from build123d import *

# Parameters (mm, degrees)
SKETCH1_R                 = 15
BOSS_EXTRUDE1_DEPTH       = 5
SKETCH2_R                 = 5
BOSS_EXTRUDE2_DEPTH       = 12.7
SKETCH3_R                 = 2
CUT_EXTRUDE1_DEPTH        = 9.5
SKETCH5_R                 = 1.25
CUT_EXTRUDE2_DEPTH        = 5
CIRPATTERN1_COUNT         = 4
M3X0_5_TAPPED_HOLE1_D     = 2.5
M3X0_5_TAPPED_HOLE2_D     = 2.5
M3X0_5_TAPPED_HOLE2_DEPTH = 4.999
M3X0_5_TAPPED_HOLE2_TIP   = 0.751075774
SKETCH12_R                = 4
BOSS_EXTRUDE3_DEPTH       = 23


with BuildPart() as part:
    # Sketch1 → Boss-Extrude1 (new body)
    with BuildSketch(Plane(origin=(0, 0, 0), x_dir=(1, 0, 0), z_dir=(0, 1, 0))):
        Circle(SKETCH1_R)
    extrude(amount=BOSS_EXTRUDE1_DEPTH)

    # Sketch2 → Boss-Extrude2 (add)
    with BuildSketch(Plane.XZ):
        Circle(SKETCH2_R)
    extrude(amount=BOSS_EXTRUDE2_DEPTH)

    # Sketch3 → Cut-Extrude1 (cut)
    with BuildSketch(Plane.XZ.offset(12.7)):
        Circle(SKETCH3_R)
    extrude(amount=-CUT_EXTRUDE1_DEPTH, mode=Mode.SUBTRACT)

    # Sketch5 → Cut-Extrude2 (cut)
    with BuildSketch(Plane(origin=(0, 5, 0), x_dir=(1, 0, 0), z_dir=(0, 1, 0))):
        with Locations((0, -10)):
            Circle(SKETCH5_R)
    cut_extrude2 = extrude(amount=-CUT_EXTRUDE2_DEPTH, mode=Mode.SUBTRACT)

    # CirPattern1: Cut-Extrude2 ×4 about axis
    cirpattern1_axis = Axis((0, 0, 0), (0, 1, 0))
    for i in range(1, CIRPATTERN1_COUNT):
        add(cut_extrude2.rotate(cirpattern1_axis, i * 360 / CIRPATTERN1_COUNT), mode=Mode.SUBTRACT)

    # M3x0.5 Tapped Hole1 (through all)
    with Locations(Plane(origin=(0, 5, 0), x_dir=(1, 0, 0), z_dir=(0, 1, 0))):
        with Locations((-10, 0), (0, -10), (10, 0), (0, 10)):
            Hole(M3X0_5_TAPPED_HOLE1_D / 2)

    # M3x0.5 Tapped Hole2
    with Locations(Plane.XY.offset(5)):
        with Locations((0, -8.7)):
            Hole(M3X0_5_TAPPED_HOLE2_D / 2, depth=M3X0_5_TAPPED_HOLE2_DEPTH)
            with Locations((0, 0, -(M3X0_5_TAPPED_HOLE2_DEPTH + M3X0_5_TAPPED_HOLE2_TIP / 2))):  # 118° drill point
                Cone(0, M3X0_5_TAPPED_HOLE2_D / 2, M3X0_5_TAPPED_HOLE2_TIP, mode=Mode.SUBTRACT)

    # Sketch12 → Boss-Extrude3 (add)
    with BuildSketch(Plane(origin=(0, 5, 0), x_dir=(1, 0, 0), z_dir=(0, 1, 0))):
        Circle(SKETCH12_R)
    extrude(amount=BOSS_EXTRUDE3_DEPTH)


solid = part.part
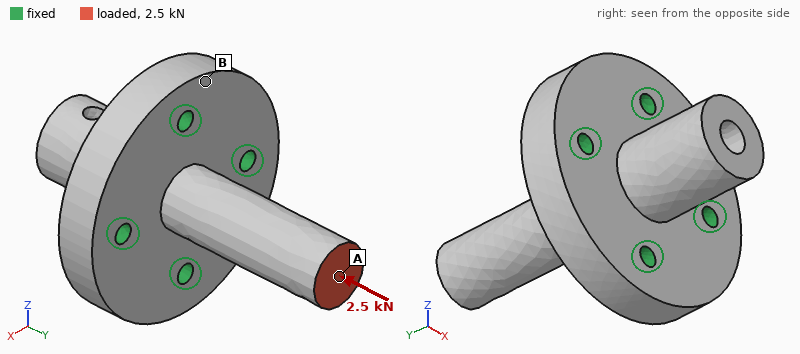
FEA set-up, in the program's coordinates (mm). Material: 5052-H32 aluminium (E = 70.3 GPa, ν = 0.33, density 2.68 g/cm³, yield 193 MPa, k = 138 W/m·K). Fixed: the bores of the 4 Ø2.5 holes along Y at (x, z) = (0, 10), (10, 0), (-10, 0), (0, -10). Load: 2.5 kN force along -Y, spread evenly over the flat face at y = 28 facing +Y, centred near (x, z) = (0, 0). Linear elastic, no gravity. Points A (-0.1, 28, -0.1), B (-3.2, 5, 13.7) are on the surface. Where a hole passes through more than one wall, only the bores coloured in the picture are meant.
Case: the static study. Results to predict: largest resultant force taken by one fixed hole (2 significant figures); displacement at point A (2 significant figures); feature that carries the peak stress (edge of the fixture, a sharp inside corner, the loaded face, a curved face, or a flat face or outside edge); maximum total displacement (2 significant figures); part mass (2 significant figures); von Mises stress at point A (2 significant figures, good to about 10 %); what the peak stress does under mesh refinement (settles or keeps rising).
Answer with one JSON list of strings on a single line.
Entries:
["630 N", "23 µm", "edge of the fixture", "23 µm", "15 g", "50 MPa", "keeps rising"]
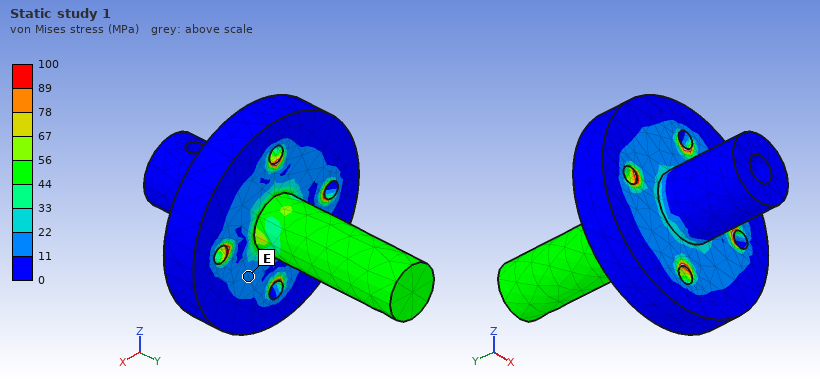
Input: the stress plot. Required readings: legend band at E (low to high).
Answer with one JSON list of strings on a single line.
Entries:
["11 to 22 MPa"]
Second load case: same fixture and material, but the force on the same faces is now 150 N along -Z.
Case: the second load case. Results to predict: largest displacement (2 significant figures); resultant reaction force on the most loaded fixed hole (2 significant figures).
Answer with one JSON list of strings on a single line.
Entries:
["61 µm", "210 N"]
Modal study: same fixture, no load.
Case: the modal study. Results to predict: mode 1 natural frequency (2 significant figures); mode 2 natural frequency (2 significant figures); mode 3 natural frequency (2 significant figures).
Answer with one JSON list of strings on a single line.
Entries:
["8600 Hz", "8600 Hz", "26 kHz"]
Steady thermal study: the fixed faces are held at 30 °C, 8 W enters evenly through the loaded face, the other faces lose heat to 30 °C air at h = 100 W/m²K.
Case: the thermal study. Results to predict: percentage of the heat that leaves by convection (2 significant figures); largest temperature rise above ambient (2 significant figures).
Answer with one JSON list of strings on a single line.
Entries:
["13 %", "28 K"]
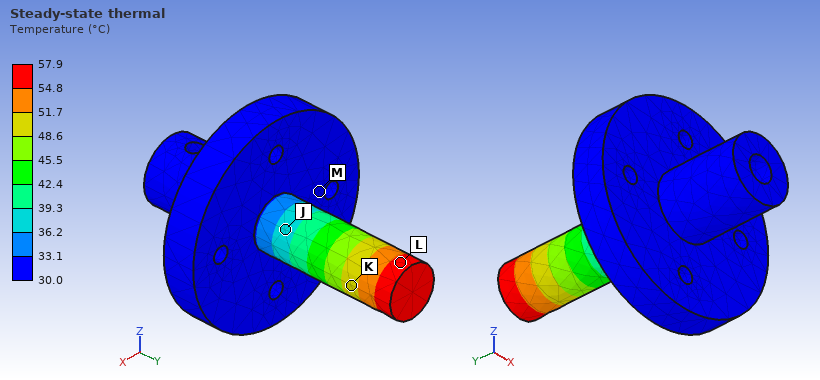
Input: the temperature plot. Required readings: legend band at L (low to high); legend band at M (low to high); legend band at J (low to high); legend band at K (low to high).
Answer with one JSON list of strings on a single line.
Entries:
["54.8 to 57.9 °C", "30.0 to 33.1 °C", "36.2 to 39.3 °C", "48.6 to 51.7 °C"]
